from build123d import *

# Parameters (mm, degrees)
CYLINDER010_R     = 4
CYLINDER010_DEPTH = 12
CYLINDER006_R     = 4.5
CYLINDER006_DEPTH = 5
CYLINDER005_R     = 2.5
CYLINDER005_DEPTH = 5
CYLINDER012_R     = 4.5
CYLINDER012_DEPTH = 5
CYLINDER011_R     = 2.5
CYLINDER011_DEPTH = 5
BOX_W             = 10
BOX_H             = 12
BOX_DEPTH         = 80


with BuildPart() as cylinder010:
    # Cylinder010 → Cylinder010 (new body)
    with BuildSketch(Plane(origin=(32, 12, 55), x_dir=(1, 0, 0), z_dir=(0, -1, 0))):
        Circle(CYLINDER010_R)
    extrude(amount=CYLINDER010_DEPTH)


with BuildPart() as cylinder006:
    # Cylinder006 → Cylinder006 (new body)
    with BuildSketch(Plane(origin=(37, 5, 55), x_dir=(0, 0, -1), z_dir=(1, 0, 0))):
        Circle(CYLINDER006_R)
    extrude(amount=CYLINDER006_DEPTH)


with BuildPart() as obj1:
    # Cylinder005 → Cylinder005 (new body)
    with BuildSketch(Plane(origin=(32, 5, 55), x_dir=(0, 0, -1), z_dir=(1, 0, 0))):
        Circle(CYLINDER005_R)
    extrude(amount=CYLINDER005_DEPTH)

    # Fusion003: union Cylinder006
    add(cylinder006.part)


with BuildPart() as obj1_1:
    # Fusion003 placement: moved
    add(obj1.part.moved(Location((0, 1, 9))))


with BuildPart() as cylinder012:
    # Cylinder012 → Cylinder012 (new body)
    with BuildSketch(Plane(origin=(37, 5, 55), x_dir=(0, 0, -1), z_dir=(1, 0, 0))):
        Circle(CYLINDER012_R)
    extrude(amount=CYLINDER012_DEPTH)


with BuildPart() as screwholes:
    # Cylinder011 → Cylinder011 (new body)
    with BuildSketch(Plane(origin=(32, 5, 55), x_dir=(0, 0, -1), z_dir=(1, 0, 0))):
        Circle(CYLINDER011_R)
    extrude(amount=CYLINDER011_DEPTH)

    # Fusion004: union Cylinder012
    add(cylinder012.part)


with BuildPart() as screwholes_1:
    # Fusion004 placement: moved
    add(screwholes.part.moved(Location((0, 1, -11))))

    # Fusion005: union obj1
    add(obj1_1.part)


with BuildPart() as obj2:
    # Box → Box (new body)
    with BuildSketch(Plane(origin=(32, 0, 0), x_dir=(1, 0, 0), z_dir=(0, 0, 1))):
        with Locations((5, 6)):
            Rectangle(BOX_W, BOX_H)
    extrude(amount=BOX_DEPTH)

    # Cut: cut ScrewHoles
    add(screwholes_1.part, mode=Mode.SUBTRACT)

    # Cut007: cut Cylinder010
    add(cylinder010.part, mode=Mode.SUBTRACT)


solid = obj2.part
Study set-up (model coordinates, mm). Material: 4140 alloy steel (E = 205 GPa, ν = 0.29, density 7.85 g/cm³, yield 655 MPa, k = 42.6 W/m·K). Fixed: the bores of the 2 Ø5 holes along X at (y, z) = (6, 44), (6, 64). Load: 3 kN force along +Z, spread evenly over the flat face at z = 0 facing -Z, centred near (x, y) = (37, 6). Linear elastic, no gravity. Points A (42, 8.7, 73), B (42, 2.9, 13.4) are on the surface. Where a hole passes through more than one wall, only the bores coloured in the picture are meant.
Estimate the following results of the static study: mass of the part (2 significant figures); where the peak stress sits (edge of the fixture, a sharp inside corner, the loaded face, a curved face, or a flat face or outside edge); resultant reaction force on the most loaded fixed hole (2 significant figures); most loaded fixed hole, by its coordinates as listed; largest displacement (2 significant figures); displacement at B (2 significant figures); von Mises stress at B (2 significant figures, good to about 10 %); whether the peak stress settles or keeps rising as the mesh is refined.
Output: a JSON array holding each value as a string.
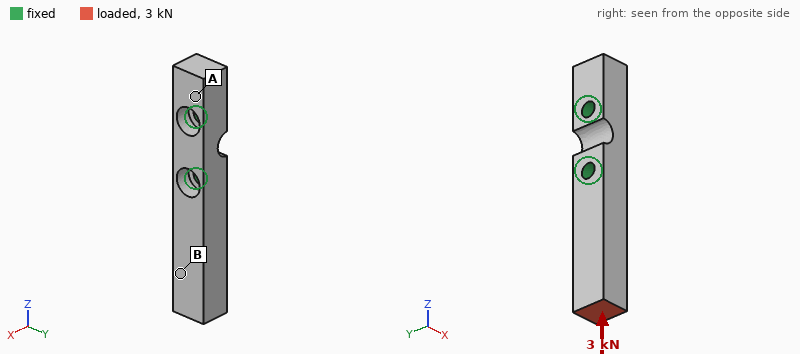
["66 g", "edge of the fixture", "2.6 kN", "(6, 44)", "20 µm", "14 µm", "25 MPa", "keeps rising"]
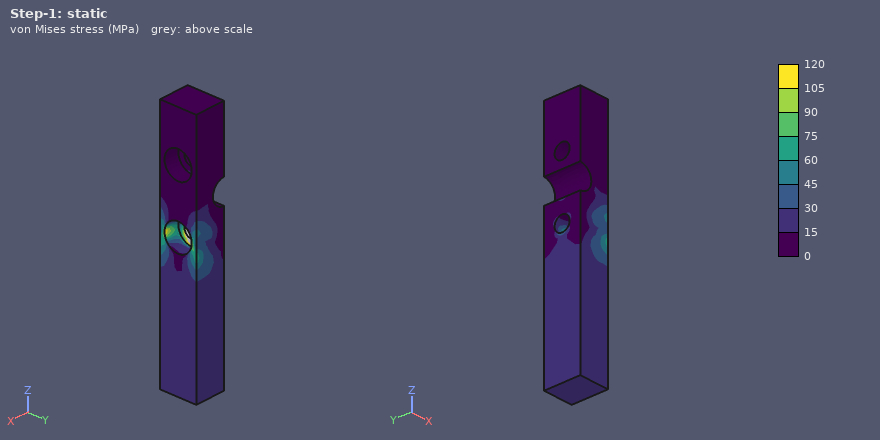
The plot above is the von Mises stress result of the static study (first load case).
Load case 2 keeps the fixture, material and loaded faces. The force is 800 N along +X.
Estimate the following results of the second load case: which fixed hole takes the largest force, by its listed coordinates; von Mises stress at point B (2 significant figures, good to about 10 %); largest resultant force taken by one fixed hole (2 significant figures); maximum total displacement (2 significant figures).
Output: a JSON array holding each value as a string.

["(6, 44)", "54 MPa", "1.9 kN", "0.18 mm"]
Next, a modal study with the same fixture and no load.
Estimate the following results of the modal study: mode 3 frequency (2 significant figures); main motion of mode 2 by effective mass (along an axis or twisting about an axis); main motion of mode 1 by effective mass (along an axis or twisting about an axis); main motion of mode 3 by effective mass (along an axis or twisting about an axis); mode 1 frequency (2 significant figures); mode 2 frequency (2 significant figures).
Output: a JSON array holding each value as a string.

["14 kHz", "along Y", "along X", "twisting about Z", "3200 Hz", "4000 Hz"]
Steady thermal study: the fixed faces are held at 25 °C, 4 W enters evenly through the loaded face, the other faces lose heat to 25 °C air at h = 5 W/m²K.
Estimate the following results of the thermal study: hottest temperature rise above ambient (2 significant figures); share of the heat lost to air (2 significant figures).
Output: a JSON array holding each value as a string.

["35 K", "4.5 %"]
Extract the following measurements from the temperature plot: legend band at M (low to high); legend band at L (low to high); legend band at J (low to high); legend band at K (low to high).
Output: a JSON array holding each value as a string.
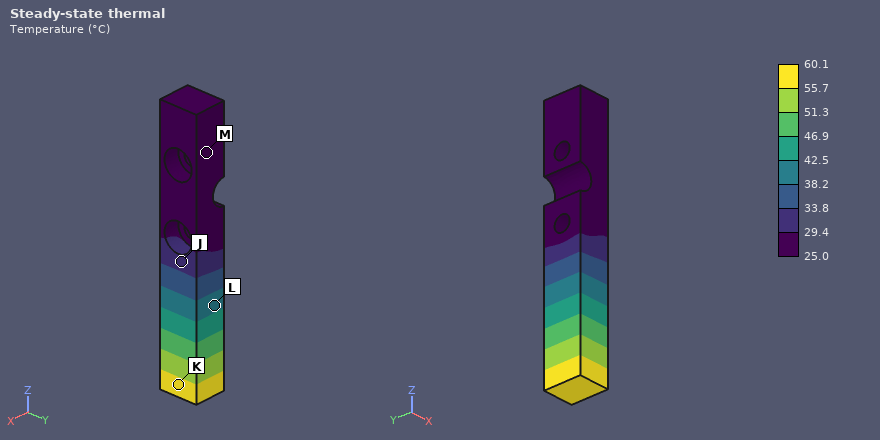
["25.0 to 29.4 °C", "38.2 to 42.5 °C", "29.4 to 33.8 °C", "55.7 to 60.1 °C"]
